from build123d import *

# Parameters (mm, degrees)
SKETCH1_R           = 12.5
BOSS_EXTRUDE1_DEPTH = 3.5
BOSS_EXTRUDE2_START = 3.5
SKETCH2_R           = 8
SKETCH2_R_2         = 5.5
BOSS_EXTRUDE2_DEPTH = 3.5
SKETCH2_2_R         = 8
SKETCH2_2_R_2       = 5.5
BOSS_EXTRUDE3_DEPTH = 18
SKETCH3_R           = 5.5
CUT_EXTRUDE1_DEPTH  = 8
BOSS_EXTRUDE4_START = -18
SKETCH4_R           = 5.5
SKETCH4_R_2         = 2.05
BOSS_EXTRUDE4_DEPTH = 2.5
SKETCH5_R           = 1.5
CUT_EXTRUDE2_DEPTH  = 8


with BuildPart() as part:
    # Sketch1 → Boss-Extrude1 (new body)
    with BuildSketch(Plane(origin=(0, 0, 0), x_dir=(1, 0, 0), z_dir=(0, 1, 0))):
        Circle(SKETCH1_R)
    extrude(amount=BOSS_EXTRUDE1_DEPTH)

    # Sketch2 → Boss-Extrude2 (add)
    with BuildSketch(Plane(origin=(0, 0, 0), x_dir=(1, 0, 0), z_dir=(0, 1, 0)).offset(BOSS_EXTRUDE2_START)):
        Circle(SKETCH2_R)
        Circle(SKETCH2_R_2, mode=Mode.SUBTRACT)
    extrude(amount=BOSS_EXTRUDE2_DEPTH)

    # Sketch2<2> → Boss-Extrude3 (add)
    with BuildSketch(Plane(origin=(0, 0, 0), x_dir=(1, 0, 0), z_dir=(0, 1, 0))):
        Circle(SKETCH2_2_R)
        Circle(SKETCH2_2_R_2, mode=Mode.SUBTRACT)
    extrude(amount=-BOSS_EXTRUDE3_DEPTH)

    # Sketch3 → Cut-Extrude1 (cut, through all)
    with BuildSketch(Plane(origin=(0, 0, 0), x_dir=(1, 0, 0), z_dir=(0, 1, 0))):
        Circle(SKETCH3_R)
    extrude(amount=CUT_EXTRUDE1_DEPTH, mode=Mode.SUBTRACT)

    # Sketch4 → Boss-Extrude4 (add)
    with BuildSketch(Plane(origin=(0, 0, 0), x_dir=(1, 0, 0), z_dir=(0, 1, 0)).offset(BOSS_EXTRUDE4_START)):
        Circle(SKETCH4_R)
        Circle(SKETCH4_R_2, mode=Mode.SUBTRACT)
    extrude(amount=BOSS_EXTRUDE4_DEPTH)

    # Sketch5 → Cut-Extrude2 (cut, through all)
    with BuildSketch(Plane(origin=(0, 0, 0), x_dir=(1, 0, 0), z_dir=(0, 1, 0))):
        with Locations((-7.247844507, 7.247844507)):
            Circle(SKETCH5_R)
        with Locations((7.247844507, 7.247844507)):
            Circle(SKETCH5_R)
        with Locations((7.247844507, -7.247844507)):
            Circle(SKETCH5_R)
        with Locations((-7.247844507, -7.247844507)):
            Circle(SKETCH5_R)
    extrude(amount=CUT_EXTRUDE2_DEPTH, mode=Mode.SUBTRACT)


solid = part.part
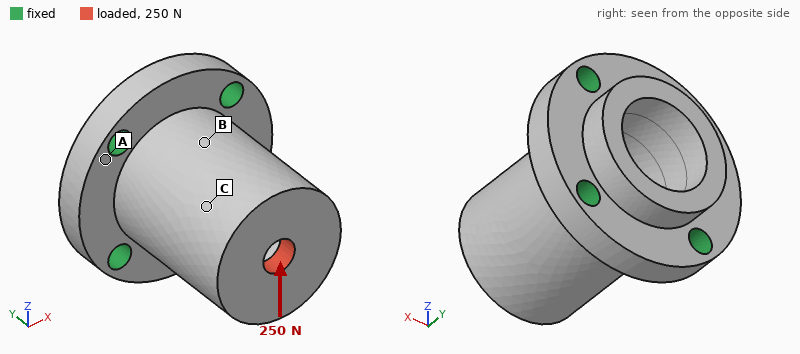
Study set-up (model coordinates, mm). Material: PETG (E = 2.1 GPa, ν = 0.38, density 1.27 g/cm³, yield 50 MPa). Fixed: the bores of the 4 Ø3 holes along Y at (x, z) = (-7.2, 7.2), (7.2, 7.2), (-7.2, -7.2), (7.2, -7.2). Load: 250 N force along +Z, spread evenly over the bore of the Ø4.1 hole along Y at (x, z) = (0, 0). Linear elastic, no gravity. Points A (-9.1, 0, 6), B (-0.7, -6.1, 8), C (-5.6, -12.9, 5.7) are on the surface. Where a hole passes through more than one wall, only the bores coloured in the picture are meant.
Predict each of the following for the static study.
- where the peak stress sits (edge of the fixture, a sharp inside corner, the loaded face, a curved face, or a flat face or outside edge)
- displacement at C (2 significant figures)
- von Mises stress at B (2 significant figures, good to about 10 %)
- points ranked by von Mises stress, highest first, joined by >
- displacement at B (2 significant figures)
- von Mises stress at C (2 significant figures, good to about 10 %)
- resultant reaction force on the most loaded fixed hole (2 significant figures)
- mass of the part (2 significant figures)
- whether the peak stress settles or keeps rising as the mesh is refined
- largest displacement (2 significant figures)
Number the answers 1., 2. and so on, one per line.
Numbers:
1. edge of the fixture
2. 0.20 mm
3. 7.5 MPa
4. B > C > A
5. 0.12 mm
6. 5.1 MPa
7. 180 N
8. 4.8 g
9. keeps rising
10. 0.30 mm
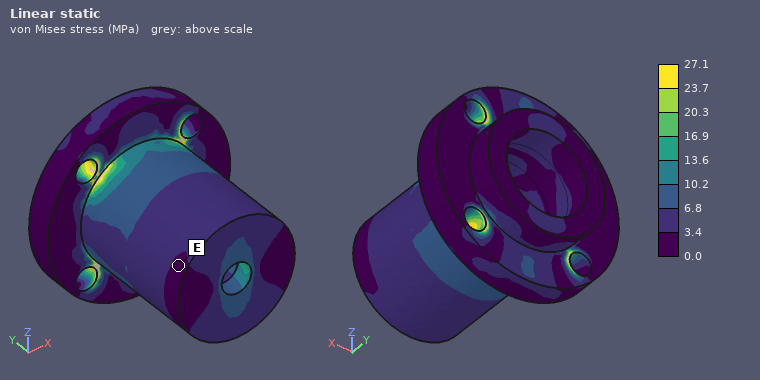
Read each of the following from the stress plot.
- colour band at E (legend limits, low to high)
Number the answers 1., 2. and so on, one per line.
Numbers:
1. 0.0 to 3.4 MPa
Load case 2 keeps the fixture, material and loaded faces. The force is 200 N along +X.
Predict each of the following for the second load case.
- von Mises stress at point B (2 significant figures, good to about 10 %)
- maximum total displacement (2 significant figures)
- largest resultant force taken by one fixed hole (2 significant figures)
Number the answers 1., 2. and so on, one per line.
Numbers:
1. 5.2 MPa
2. 0.24 mm
3. 140 N
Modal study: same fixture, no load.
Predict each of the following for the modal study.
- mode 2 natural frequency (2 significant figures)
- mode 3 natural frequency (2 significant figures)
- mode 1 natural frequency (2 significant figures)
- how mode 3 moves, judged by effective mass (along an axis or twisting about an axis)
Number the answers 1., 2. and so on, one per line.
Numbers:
1. 4400 Hz
2. 9400 Hz
3. 4400 Hz
4. twisting about Y
